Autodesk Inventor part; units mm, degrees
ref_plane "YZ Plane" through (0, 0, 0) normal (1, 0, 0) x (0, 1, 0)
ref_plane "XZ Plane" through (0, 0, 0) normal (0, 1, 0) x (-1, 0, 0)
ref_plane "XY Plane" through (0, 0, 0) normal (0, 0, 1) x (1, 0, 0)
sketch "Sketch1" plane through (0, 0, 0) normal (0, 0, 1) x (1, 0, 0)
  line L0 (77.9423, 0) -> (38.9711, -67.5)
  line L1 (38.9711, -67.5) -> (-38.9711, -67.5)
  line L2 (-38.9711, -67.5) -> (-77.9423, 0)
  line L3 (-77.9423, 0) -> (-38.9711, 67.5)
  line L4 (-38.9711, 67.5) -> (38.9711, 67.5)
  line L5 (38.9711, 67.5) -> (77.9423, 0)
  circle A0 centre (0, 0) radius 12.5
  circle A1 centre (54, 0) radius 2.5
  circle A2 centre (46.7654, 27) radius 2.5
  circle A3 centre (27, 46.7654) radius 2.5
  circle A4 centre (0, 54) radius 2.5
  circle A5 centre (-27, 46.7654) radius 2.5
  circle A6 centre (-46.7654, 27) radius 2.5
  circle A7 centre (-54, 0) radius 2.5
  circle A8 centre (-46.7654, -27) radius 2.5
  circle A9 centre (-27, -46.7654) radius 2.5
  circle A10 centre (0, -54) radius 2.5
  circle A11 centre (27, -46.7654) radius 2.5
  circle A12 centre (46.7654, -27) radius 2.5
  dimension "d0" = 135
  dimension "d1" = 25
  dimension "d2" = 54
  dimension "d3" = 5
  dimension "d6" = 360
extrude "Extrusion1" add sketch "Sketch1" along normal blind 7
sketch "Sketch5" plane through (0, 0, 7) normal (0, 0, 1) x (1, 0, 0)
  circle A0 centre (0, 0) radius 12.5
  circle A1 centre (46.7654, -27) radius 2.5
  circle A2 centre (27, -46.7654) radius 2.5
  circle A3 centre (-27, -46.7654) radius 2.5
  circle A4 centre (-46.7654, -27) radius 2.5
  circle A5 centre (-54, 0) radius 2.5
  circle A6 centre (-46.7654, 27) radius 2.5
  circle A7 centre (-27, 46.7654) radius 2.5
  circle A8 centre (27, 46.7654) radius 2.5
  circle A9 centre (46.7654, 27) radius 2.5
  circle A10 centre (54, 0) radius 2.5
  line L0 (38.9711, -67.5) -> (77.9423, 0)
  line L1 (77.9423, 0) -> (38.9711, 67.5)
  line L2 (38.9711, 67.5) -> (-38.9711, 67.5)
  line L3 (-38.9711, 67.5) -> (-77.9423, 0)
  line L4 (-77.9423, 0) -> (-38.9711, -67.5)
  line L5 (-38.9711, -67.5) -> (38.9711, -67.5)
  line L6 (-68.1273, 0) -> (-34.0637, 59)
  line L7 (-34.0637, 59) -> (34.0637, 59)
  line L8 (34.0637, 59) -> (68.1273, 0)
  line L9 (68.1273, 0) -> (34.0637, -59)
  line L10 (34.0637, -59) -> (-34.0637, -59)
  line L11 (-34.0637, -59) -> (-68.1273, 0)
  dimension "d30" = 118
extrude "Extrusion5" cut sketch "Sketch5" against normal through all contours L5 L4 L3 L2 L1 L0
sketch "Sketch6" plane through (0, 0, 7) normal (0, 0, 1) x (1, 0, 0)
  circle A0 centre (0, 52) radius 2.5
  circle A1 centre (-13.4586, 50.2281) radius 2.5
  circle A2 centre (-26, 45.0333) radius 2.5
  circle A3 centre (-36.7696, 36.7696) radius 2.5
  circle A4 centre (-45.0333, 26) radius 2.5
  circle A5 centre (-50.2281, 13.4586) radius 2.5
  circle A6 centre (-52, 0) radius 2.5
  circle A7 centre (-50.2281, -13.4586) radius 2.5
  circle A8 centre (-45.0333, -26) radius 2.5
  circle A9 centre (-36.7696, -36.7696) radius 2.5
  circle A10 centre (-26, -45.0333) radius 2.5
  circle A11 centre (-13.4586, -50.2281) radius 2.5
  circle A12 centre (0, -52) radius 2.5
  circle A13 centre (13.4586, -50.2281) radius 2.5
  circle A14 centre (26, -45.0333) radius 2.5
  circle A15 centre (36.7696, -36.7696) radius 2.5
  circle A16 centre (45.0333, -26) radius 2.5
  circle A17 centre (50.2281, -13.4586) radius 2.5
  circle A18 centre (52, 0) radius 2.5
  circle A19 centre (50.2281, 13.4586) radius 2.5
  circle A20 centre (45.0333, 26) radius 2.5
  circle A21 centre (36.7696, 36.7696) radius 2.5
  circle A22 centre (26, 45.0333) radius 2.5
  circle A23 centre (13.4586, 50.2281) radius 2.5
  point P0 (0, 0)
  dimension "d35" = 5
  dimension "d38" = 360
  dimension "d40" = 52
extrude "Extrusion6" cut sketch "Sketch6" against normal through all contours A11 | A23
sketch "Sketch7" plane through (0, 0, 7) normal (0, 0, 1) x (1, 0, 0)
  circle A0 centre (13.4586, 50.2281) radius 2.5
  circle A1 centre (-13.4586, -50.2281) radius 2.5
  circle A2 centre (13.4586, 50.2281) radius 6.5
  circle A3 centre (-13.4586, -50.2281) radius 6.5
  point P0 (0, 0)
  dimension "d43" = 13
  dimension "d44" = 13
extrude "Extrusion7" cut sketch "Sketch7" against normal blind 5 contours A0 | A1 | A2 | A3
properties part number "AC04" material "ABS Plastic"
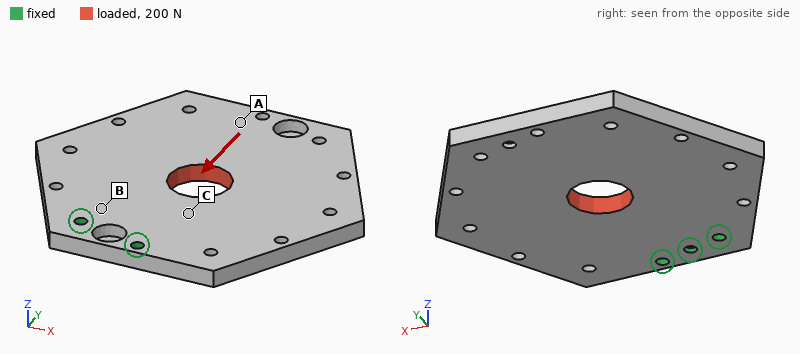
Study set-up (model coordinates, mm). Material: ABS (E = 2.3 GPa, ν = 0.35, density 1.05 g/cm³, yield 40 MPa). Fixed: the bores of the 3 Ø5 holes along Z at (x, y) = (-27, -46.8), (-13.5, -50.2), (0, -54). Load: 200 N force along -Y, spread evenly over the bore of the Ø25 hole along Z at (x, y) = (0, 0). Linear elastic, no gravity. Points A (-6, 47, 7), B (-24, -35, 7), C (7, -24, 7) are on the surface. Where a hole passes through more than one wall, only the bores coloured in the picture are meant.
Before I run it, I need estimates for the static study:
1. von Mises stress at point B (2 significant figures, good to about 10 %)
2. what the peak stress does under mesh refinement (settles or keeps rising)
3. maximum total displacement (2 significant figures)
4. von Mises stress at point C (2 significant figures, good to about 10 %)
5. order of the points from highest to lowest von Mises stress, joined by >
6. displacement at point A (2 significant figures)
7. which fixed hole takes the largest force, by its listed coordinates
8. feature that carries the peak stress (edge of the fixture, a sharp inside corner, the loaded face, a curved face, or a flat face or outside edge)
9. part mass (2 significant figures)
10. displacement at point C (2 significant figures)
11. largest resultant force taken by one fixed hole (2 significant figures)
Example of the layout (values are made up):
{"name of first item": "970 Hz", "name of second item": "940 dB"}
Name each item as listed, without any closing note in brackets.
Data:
{"von Mises stress at point B": "0.35 MPa", "what the peak stress does under mesh refinement": "keeps rising", "maximum total displacement": "69 µm", "von Mises stress at point C": "0.69 MPa", "order of the points from highest to lowest von Mises stress, joined by >": "C > B > A", "displacement at point A": "58 µm", "which fixed hole takes the largest force, by its listed coordinates": "(0, -54)", "feature that carries the peak stress": "edge of the fixture", "part mass": "82 g", "displacement at point C": "24 µm", "largest resultant force taken by one fixed hole": "170 N"}
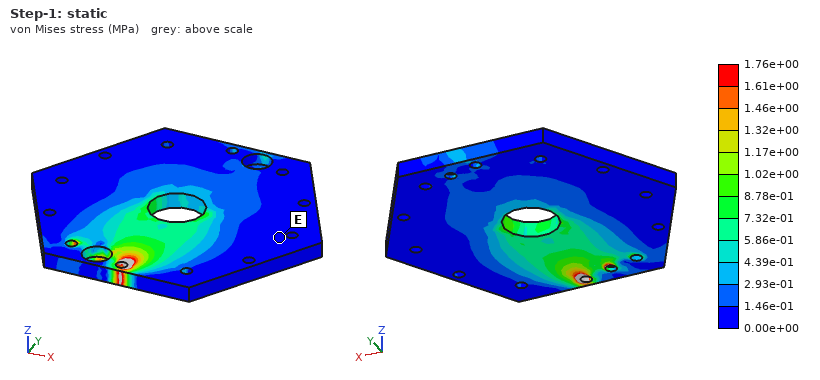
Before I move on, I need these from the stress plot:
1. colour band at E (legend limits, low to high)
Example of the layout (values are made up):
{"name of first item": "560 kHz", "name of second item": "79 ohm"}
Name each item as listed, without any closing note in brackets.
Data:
{"colour band at E": "0.00e+00 to 1.46e-01 MPa"}
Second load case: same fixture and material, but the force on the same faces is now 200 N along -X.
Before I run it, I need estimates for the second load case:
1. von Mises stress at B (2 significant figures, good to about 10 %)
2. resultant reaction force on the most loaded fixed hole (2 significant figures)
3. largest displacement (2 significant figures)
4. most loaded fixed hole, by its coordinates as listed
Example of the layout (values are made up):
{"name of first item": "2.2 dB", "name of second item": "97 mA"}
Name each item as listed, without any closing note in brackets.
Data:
{"von Mises stress at B": "2.0 MPa", "resultant reaction force on the most loaded fixed hole": "350 N", "largest displacement": "0.23 mm", "most loaded fixed hole, by its coordinates as listed": "(-27, -46.8)"}
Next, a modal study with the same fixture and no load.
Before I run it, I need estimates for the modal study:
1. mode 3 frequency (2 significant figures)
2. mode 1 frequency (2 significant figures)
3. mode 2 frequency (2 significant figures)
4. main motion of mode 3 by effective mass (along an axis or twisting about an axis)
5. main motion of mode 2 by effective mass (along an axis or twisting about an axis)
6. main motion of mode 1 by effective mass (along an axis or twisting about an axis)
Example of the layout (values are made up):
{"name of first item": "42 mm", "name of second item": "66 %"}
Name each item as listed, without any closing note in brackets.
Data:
{"mode 3 frequency": "580 Hz", "mode 1 frequency": "120 Hz", "mode 2 frequency": "260 Hz", "main motion of mode 3 by effective mass": "along X", "main motion of mode 2 by effective mass": "twisting about Y", "main motion of mode 1 by effective mass": "along Z"}
